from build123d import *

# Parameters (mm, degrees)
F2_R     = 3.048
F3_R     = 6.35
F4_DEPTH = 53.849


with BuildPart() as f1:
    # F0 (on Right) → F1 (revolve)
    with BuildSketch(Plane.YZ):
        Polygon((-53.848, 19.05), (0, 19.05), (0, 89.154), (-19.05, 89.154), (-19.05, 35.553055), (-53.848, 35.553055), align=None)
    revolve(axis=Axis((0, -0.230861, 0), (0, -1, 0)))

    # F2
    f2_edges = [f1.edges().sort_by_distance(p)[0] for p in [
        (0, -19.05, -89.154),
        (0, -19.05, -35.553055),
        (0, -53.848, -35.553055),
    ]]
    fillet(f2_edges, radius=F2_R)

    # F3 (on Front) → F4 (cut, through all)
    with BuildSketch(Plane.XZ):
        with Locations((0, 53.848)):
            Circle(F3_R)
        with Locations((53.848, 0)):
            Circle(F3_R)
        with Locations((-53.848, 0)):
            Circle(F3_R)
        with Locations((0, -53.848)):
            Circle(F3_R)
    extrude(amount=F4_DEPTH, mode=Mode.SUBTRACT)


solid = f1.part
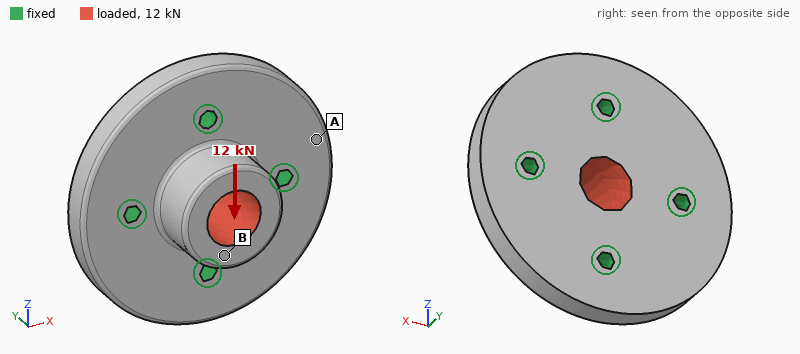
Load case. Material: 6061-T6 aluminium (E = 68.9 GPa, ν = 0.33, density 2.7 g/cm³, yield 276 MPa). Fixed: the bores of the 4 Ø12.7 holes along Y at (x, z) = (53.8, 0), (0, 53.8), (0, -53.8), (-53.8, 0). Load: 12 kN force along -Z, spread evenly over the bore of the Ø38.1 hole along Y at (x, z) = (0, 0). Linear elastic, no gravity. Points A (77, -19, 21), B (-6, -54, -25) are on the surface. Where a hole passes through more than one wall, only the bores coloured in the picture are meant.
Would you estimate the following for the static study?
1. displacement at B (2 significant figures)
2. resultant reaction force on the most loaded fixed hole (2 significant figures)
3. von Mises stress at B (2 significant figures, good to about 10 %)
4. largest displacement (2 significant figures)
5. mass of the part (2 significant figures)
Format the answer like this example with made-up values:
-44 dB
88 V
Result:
9.2 µm
4.3 kN
3.9 MPa
9.4 µm
1.5 kg
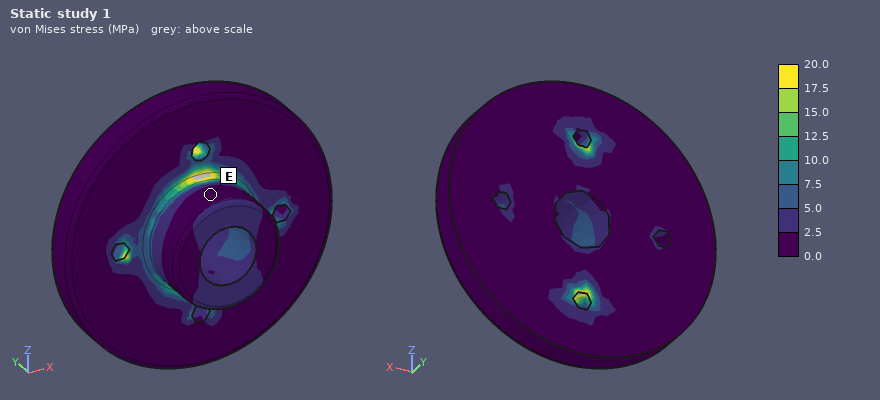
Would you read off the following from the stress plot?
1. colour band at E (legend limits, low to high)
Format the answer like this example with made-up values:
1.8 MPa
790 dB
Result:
0.0 to 2.5 MPa
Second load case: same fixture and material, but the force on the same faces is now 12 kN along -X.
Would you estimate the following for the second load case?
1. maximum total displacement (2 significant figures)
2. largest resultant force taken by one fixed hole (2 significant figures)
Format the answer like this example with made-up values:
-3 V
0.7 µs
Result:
9.3 µm
4.3 kN
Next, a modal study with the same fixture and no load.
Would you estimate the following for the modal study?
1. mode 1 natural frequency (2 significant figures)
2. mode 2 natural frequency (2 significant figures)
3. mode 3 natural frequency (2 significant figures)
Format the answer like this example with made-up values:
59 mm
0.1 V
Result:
5800 Hz
6300 Hz
6300 Hz
